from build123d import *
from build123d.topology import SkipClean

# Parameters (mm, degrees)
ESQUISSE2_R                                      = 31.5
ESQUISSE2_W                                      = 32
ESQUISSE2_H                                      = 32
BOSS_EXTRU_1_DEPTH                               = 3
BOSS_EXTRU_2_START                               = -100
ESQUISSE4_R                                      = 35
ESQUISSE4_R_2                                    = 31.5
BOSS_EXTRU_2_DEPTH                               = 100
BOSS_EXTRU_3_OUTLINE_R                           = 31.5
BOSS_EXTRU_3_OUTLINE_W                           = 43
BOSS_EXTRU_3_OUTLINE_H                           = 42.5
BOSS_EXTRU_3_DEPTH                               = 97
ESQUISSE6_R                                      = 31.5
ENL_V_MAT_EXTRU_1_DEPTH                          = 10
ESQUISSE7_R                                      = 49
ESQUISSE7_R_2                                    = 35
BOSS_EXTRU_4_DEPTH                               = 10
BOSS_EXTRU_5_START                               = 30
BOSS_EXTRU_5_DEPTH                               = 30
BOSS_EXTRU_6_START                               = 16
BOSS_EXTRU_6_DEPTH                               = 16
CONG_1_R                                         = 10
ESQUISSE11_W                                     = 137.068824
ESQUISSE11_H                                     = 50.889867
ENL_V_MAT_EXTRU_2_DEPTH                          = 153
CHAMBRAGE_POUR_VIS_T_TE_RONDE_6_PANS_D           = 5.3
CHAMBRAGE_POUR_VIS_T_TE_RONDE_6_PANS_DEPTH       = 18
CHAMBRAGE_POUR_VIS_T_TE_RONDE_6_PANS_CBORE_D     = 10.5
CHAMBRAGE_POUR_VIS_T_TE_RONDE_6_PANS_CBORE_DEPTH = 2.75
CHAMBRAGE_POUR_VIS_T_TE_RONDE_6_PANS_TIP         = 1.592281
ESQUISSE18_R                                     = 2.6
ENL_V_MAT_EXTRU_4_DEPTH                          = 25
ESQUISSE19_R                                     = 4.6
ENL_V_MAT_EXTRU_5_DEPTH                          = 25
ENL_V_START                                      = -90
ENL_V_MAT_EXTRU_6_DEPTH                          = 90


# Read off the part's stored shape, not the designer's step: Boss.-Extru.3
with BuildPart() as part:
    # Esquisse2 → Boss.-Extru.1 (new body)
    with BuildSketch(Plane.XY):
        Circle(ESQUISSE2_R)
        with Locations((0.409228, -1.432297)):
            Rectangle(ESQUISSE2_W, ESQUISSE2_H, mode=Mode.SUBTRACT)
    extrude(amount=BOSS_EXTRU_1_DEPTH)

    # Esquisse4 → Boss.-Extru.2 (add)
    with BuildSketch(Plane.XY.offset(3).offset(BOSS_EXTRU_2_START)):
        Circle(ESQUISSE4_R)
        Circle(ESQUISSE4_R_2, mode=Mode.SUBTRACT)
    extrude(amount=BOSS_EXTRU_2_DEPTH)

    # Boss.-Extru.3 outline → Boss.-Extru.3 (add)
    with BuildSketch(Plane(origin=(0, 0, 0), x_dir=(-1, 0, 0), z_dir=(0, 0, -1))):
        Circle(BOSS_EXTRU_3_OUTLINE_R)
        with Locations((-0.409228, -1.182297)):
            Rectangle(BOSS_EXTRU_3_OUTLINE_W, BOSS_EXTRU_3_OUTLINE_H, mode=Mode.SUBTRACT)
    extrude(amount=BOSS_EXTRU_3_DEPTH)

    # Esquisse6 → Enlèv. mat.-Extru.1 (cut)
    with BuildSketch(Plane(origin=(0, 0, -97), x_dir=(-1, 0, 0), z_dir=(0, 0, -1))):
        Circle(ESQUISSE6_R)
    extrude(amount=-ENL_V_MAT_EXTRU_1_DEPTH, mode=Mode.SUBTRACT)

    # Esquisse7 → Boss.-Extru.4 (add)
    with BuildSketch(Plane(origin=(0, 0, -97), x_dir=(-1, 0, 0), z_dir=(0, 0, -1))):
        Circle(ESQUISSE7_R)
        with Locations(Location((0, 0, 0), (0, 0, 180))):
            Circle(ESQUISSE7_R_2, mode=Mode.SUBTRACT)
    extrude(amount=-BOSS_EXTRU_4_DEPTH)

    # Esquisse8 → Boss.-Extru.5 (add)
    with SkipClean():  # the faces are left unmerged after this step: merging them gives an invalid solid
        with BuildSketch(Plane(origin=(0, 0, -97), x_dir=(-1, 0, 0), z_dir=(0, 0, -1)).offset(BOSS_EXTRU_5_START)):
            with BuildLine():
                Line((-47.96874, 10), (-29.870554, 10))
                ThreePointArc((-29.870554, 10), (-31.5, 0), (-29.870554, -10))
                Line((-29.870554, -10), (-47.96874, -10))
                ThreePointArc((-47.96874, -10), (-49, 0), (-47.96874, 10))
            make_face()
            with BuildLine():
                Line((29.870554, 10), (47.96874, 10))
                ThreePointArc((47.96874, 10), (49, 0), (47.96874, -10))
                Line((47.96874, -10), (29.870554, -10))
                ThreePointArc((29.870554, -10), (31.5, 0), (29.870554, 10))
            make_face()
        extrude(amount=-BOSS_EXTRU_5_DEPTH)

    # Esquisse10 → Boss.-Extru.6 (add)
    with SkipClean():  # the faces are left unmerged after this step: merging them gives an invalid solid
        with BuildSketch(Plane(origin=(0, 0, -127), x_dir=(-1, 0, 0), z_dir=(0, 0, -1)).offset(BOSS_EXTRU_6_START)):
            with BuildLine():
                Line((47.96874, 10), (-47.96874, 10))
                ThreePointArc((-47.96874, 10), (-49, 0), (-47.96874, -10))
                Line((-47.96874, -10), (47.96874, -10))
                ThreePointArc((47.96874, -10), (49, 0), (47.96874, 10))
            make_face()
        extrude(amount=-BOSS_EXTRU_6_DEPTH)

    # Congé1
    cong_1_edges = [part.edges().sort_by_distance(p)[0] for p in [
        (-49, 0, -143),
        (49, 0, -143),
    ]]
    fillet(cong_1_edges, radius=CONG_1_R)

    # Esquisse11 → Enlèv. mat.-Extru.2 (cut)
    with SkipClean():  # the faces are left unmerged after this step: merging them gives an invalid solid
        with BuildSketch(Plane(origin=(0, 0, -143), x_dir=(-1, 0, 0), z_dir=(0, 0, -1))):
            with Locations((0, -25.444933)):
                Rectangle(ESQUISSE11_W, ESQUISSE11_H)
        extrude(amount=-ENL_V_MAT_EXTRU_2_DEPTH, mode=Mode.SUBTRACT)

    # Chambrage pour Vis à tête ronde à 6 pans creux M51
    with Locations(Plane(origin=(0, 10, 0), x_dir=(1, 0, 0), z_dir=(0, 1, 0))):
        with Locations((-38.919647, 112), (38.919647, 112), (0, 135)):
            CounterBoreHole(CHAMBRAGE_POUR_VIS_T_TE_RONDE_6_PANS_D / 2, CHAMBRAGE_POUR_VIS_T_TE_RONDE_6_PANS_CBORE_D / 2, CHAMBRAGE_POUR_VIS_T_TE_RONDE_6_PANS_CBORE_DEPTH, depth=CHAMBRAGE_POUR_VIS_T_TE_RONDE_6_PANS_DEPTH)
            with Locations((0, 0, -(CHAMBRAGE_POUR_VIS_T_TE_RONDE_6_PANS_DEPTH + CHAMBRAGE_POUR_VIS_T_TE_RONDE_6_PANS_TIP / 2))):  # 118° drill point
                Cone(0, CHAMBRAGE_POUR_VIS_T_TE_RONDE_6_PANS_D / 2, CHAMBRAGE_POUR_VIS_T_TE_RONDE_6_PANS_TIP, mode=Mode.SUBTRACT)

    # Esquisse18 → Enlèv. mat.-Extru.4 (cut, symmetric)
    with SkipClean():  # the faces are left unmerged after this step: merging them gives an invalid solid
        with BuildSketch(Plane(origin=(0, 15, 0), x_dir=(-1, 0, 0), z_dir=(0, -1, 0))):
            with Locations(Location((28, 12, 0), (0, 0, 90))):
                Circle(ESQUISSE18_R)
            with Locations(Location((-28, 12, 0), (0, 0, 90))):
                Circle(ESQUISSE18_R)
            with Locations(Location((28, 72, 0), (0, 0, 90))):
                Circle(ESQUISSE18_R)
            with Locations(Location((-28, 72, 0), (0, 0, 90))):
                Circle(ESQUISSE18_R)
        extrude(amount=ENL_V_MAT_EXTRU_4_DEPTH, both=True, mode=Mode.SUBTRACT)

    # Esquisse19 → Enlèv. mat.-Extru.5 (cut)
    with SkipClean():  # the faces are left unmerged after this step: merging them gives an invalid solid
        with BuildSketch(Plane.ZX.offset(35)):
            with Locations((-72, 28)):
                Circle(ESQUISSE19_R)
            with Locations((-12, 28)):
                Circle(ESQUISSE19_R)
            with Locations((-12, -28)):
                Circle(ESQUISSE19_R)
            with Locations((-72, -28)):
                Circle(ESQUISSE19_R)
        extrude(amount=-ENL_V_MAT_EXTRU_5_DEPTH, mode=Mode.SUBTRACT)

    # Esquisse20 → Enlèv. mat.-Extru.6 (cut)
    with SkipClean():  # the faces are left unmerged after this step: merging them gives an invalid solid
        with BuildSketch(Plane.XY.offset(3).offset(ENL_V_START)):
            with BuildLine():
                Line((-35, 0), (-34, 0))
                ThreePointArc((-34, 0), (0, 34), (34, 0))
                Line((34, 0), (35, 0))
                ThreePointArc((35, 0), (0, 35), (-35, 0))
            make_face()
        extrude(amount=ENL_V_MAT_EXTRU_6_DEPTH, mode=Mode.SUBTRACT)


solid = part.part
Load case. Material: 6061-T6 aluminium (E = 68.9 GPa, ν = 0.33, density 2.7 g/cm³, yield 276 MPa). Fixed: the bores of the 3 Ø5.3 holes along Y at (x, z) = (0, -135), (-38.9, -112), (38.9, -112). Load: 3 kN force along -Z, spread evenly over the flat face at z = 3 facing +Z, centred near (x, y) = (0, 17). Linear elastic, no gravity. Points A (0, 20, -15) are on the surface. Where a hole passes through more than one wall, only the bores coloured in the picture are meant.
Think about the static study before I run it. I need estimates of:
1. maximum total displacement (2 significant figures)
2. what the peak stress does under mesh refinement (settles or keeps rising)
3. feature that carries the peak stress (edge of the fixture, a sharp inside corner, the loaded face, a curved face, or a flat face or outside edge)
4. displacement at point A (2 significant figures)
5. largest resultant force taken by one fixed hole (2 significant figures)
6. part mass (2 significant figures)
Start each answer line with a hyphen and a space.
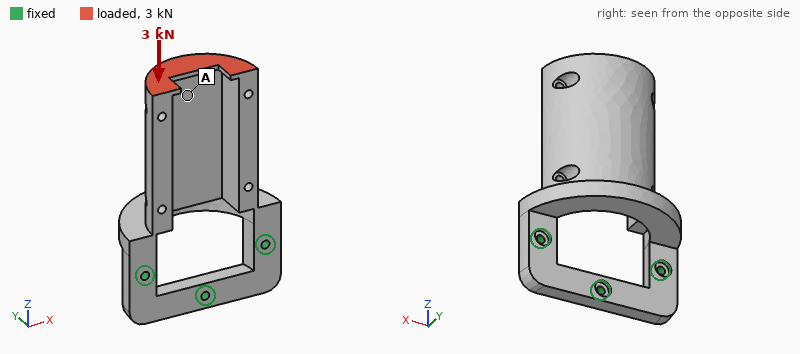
- 0.57 mm
- keeps rising
- edge of the fixture
- 0.47 mm
- 1.5 kN
- 350 g
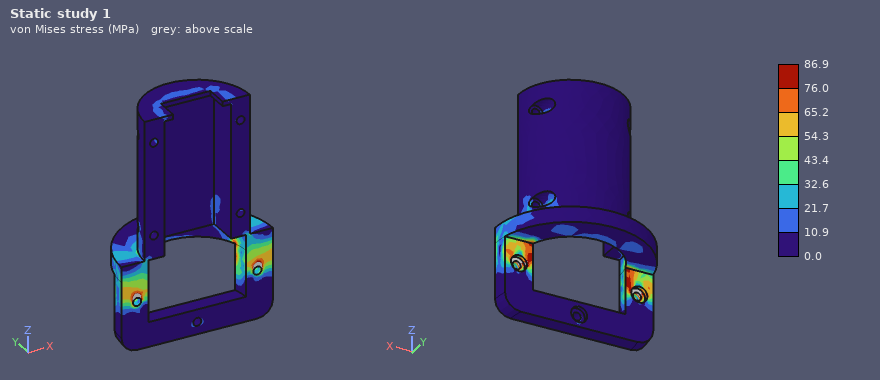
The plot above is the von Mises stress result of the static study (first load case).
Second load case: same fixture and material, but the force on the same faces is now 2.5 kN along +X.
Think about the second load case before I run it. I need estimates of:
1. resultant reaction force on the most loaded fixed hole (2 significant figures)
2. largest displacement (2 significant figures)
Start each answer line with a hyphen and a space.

- 3.8 kN
- 0.34 mm
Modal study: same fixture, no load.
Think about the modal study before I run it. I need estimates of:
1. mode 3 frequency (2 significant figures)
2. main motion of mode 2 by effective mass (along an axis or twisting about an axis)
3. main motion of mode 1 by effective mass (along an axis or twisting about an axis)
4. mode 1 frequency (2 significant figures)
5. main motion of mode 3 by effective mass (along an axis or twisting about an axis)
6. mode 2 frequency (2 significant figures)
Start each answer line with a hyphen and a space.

- 2800 Hz
- along X
- along Y
- 390 Hz
- along X
- 1600 Hz
